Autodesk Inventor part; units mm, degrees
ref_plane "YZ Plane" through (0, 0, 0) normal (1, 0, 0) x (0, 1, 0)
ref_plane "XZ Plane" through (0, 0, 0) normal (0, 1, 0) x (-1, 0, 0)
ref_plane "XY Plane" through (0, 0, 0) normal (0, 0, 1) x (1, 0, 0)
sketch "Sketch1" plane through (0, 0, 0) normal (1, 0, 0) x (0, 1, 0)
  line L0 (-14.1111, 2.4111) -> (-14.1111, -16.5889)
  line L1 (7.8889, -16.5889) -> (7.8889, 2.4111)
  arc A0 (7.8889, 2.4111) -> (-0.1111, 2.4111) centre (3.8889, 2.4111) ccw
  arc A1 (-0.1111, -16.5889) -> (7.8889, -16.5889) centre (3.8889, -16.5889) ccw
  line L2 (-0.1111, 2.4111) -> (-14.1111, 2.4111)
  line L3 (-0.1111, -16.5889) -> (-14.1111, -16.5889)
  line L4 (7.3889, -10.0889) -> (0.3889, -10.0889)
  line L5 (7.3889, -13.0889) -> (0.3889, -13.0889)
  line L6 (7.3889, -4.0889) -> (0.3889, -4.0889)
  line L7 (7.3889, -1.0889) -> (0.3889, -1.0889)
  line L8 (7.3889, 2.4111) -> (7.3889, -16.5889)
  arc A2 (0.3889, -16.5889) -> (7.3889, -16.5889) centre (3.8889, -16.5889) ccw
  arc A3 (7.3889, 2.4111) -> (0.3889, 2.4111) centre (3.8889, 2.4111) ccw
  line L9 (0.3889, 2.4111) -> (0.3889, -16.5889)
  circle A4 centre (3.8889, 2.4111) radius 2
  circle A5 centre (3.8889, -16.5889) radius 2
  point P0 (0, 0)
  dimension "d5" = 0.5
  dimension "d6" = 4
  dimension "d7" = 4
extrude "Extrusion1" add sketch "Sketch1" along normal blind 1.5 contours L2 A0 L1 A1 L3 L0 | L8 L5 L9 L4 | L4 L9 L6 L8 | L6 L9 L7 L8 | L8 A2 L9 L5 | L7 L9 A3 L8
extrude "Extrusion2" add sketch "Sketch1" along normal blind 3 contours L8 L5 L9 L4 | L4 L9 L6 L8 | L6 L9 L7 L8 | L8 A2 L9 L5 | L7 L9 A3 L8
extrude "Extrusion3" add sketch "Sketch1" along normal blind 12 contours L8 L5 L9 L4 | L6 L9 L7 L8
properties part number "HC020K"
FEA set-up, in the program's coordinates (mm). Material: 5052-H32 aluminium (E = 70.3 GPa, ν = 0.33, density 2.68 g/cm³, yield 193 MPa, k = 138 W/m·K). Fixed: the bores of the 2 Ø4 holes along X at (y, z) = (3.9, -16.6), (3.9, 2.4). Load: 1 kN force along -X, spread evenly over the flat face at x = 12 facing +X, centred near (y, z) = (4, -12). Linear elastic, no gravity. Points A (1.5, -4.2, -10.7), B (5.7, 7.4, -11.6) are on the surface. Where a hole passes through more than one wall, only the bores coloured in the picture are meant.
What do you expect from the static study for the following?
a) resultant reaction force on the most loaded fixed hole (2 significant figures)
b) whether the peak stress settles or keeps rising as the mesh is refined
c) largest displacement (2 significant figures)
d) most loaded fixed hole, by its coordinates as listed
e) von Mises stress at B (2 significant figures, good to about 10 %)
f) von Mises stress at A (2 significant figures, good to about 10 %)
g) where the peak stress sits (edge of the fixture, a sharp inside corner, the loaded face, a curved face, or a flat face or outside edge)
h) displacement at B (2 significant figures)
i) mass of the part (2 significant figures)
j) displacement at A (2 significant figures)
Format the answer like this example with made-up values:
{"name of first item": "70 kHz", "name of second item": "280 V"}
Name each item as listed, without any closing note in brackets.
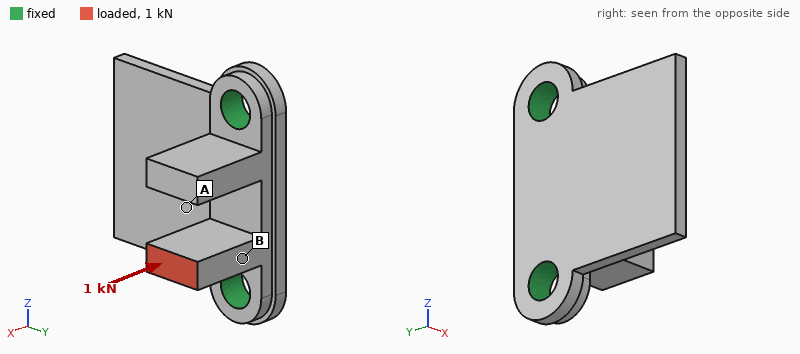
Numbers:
{"resultant reaction force on the most loaded fixed hole": "840 N", "whether the peak stress settles or keeps rising as the mesh is refined": "keeps rising", "largest displacement": "28 µm", "most loaded fixed hole, by its coordinates as listed": "(3.9, -16.6)", "von Mises stress at B": "45 MPa", "von Mises stress at A": "15 MPa", "where the peak stress sits": "edge of the fixture", "displacement at B": "14 µm", "mass of the part": "3.4 g", "displacement at A": "9.4 µm"}
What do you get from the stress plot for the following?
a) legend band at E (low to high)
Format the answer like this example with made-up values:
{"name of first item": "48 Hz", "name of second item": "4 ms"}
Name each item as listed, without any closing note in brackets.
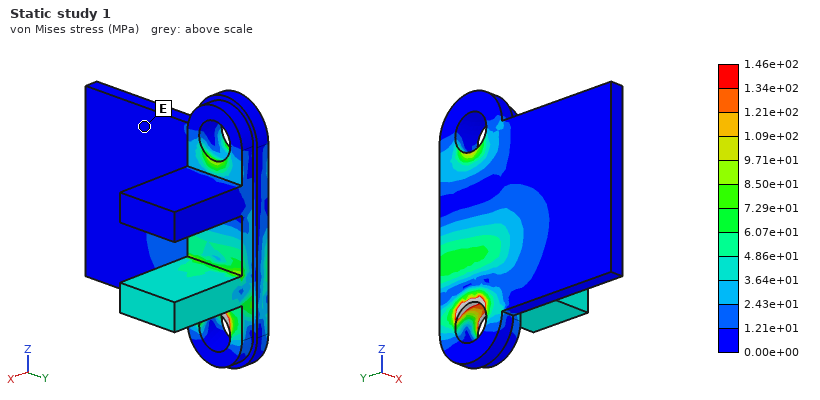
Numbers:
{"legend band at E": "0.00e+00 to 1.21e+01 MPa"}
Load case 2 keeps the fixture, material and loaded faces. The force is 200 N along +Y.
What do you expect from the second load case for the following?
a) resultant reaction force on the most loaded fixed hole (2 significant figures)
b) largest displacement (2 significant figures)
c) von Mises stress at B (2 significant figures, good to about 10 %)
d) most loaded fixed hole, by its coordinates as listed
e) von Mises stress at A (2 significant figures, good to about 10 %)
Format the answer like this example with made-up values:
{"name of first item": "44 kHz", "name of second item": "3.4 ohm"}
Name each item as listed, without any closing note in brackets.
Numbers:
{"resultant reaction force on the most loaded fixed hole": "170 N", "largest displacement": "43 µm", "von Mises stress at B": "52 MPa", "most loaded fixed hole, by its coordinates as listed": "(3.9, -16.6)", "von Mises stress at A": "13 MPa"}
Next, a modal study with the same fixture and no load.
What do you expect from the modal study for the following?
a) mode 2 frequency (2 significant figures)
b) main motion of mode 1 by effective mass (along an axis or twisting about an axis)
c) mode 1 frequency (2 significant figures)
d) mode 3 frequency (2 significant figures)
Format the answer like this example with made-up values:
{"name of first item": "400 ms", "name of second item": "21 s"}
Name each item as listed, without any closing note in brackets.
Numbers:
{"mode 2 frequency": "11 kHz", "main motion of mode 1 by effective mass": "along X", "mode 1 frequency": "5200 Hz", "mode 3 frequency": "18 kHz"}
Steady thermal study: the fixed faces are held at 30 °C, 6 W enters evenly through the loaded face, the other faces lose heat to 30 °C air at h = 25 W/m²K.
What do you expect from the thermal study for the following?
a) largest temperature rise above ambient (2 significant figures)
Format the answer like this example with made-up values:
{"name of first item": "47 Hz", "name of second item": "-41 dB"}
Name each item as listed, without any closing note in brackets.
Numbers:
{"largest temperature rise above ambient": "24 K"}
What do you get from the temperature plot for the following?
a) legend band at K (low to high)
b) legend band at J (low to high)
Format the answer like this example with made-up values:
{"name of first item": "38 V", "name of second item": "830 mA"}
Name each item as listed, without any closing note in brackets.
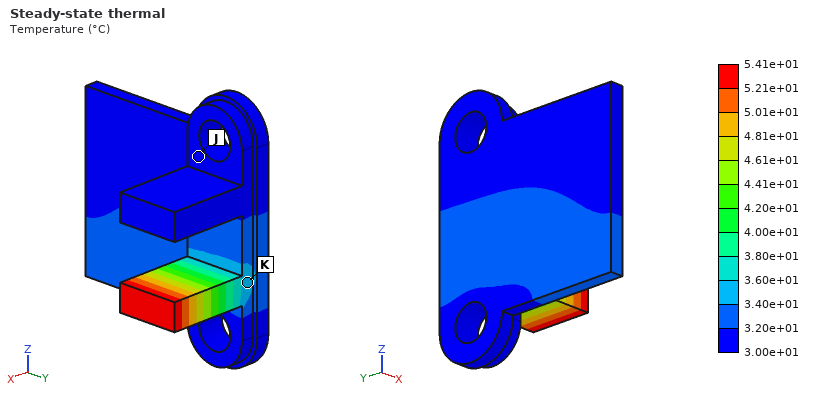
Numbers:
{"legend band at K": "3.40e+01 to 3.60e+01 °C", "legend band at J": "3.00e+01 to 3.20e+01 °C"}
